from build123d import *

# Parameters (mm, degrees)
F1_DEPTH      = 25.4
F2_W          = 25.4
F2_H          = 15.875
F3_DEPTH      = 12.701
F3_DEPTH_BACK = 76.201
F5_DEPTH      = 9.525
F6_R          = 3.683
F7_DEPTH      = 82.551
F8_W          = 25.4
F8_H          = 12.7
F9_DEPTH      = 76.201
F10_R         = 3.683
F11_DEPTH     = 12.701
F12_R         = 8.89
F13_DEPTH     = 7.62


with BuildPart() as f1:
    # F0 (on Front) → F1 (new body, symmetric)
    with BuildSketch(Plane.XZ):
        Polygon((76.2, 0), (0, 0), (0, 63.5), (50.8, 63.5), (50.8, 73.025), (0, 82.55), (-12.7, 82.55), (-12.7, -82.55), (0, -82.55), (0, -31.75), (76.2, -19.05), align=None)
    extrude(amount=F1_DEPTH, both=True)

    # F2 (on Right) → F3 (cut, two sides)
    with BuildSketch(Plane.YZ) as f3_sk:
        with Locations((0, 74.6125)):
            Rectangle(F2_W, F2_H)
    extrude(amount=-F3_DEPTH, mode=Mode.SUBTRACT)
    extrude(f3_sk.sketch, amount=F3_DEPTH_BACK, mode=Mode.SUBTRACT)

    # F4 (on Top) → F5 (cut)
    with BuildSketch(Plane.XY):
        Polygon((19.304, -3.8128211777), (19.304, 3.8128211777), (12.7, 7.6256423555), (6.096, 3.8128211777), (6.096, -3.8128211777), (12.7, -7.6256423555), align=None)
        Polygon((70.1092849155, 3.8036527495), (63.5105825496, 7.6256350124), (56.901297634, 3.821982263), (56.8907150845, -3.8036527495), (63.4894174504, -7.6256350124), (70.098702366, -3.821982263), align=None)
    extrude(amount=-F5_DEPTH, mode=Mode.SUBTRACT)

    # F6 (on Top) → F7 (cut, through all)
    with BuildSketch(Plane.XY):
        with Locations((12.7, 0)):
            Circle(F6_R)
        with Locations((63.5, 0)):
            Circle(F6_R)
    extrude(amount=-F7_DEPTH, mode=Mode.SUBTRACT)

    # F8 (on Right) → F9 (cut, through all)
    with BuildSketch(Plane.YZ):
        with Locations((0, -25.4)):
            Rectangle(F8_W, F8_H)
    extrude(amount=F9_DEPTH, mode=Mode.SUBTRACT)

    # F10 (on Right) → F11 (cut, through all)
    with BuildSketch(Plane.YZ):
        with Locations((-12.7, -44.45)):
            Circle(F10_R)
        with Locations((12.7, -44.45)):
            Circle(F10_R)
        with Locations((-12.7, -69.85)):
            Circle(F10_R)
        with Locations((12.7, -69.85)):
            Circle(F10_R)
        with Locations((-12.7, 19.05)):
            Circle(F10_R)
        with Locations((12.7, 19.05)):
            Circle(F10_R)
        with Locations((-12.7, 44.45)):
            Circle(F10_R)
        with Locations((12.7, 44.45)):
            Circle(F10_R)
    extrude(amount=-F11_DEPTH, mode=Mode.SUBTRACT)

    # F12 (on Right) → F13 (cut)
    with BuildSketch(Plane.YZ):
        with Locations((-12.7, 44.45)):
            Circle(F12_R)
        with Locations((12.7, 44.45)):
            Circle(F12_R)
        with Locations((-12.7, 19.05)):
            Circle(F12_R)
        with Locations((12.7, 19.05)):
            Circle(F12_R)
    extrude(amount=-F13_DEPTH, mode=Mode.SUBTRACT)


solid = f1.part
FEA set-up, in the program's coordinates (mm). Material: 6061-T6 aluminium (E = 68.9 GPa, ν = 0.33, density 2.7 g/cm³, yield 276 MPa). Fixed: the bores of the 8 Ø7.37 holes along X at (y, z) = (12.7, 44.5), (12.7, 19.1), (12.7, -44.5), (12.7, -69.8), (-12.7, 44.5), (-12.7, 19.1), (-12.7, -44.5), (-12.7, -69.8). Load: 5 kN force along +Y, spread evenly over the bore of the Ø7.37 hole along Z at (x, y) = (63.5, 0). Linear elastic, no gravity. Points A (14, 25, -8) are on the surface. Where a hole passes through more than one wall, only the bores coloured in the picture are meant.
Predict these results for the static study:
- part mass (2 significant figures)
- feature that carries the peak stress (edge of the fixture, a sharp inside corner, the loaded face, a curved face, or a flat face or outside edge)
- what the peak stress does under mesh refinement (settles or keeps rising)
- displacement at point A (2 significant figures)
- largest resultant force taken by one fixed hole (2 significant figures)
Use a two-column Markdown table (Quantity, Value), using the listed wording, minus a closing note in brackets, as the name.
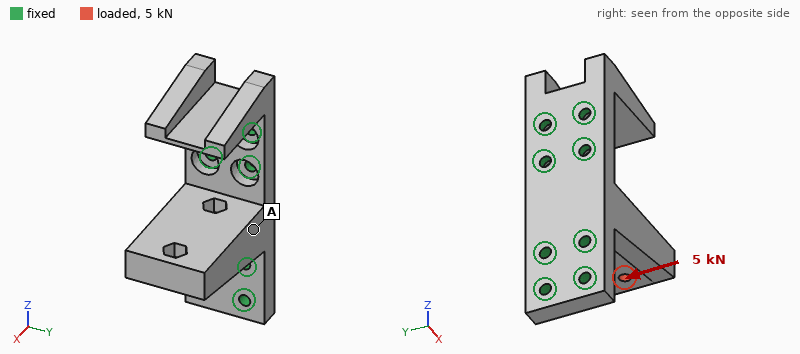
| Quantity | Value |
|---|---|
| part mass | 530 g |
| feature that carries the peak stress | edge of the fixture |
| what the peak stress does under mesh refinement | keeps rising |
| displacement at point A | 0.090 mm |
| largest resultant force taken by one fixed hole | 7.3 kN |
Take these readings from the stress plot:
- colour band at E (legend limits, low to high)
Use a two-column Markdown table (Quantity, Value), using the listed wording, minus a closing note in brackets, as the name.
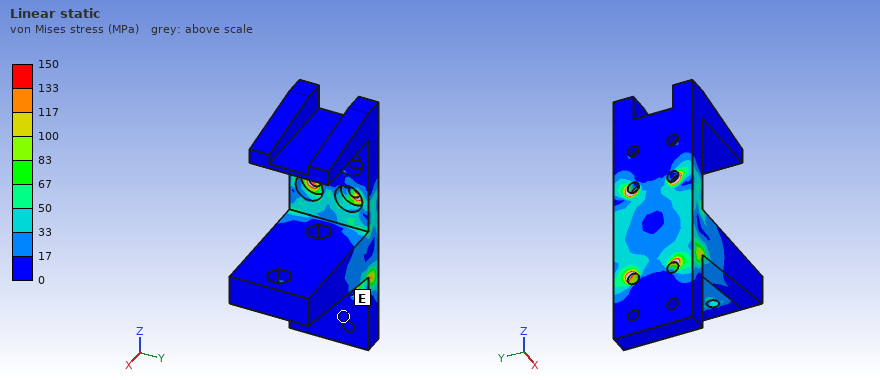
| Quantity | Value |
|---|---|
| colour band at E | 0 to 17 MPa |
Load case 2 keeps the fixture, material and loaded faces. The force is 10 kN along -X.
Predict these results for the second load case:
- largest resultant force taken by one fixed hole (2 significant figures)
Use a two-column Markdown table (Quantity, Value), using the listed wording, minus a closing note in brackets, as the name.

| Quantity | Value |
|---|---|
| largest resultant force taken by one fixed hole | 3.3 kN |
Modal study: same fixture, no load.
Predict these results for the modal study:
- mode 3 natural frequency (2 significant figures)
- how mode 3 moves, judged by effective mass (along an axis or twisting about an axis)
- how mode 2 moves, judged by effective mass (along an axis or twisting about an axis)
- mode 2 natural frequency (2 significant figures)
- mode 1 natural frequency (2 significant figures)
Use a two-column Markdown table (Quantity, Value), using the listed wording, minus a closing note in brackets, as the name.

| Quantity | Value |
|---|---|
| mode 3 natural frequency | 2600 Hz |
| how mode 3 moves, judged by effective mass | along Z |
| how mode 2 moves, judged by effective mass | along Y |
| mode 2 natural frequency | 2300 Hz |
| mode 1 natural frequency | 1700 Hz |
